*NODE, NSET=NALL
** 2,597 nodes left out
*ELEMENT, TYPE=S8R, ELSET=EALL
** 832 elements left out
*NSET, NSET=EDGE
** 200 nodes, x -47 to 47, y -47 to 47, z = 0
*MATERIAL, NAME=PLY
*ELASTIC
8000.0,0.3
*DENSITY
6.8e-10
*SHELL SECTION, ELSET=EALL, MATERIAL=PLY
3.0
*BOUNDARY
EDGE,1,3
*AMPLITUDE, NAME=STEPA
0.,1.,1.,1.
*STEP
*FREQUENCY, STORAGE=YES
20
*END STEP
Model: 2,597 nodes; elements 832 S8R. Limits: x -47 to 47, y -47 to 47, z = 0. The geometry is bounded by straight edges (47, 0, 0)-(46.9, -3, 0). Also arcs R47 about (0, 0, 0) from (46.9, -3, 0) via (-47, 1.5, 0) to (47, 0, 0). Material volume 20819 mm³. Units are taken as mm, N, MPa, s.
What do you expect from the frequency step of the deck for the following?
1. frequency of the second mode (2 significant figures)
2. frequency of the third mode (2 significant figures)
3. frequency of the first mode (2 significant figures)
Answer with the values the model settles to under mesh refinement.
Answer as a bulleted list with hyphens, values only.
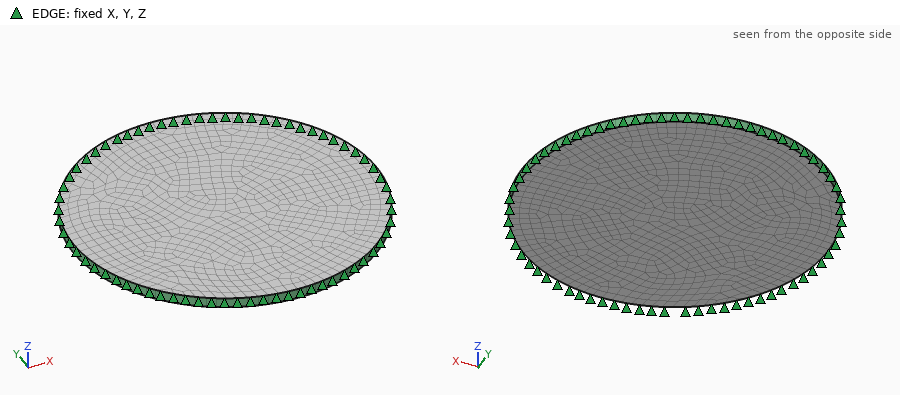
- 3100 Hz
- 3100 Hz
- 1100 Hz
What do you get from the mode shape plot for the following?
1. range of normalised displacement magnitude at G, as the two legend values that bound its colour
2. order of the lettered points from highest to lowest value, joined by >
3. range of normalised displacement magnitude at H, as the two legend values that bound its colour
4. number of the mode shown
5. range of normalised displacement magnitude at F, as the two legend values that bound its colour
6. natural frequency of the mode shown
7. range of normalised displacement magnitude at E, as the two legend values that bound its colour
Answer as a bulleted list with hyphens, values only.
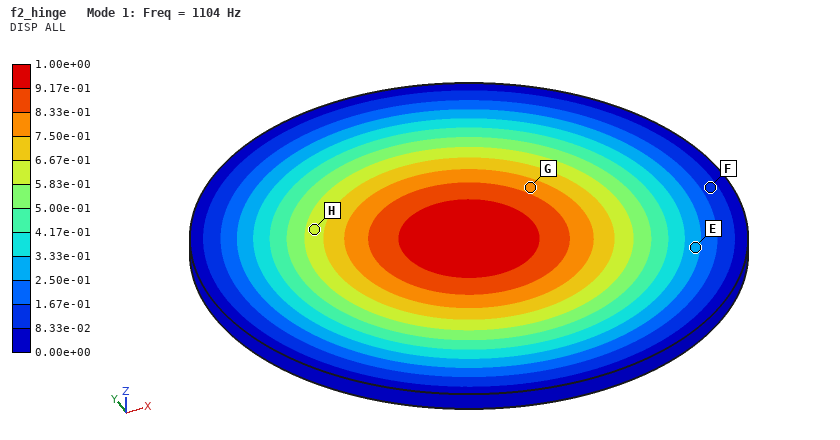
- 7.50e-01 to 8.33e-01
- G > H > E > F
- 5.83e-01 to 6.67e-01
- 1
- 8.33e-02 to 1.67e-01
- 1104 Hz
- 2.50e-01 to 3.33e-01
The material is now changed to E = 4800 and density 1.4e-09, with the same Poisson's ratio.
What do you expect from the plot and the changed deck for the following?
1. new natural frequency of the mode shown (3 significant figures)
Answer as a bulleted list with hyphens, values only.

- 596 Hz
